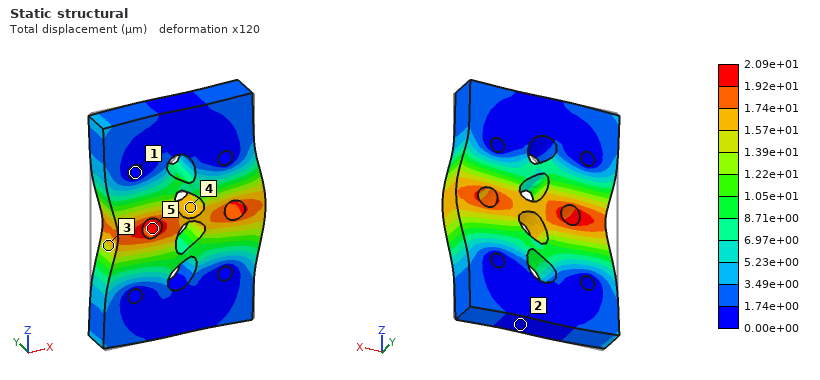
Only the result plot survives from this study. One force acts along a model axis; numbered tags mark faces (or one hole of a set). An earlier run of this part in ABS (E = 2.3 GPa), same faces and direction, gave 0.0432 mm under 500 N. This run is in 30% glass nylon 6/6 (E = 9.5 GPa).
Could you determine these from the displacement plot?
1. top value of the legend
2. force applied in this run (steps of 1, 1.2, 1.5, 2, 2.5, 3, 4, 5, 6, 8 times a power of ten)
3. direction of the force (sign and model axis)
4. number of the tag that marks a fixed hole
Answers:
2.09e+01 µm
1 kN
+X
1
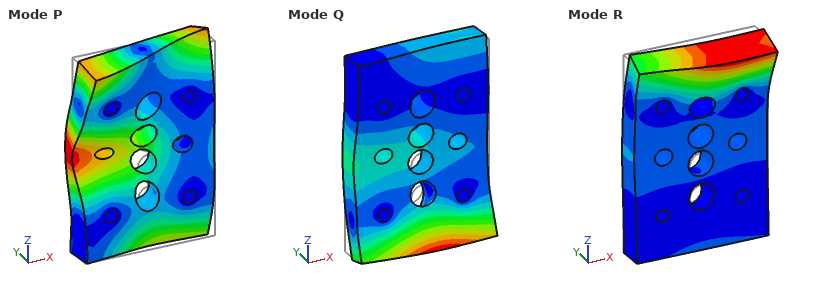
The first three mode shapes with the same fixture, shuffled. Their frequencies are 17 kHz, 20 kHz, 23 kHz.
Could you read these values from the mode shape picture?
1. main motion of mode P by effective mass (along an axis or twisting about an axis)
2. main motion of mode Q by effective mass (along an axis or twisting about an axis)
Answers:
along Y
twisting about X
